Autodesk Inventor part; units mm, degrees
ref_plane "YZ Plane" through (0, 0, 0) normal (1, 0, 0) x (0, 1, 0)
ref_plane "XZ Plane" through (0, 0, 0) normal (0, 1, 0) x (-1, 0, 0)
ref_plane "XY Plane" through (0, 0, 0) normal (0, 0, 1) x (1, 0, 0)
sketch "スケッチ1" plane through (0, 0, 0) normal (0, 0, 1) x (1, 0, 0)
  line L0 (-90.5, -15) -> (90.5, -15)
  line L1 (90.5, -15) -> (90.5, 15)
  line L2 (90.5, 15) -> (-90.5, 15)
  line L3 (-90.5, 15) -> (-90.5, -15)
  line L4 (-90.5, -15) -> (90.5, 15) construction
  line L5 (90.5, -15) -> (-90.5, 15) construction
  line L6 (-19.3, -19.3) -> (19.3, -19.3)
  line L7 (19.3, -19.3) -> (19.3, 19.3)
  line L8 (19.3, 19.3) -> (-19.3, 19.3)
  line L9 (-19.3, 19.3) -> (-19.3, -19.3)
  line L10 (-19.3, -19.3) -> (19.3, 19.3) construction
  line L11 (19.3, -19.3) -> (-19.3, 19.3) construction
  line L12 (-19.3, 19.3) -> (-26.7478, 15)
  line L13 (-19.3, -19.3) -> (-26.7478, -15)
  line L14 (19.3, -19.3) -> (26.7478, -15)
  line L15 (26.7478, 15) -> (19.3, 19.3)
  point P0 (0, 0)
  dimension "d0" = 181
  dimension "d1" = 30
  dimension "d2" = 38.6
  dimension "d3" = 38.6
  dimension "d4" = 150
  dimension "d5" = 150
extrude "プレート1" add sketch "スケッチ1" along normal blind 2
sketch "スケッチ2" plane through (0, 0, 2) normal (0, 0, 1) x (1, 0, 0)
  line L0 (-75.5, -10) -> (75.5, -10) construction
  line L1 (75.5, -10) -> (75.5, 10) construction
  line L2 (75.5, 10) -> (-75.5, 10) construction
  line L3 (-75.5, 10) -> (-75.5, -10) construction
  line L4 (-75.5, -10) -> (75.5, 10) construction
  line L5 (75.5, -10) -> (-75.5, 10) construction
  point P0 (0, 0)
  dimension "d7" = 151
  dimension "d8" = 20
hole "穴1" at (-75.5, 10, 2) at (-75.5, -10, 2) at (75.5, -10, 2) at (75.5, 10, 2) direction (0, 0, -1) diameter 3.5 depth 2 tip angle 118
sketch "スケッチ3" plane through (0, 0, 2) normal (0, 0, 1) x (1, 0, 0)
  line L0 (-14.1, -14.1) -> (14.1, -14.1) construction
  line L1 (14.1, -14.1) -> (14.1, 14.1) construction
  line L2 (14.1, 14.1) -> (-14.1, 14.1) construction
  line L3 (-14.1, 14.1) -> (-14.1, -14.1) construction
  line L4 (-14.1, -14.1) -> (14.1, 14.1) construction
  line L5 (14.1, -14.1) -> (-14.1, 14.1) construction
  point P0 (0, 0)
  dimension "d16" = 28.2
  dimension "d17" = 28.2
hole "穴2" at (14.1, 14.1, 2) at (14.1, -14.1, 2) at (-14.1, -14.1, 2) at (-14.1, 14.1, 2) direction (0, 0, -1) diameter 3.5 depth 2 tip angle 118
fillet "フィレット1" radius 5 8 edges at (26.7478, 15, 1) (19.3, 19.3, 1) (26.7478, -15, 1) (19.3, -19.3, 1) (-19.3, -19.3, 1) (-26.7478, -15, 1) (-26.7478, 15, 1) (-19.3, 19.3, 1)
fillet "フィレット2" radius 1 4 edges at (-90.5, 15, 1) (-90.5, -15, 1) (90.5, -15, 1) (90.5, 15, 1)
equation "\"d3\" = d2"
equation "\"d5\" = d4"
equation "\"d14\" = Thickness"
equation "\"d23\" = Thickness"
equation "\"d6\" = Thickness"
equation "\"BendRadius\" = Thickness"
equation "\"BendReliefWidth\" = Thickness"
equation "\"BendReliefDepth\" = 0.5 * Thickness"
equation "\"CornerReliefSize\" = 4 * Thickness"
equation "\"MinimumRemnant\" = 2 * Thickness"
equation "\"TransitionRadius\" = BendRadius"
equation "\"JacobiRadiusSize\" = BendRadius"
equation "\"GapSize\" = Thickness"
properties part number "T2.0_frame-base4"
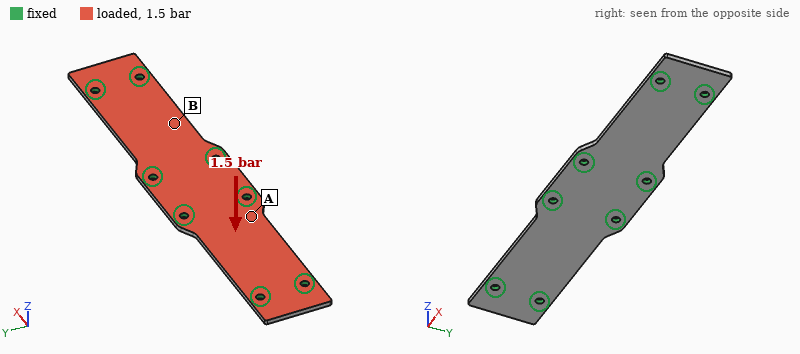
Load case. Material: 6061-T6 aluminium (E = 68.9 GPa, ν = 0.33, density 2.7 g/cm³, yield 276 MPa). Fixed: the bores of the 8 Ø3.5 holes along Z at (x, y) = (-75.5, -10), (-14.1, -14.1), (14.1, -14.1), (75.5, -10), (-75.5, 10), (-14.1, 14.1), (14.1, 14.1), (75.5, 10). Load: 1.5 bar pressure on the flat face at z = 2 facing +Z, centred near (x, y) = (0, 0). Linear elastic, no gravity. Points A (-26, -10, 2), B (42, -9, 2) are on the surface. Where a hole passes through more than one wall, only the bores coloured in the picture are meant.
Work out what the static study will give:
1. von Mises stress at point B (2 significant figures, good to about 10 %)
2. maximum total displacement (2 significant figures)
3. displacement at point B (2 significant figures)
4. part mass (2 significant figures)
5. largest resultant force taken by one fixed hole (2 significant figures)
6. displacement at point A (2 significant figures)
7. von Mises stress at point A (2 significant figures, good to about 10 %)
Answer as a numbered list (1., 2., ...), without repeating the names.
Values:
1. 31 MPa
2. 0.11 mm
3. 0.11 mm
4. 31 g
5. 110 N
6. 0.046 mm
7. 11 MPa
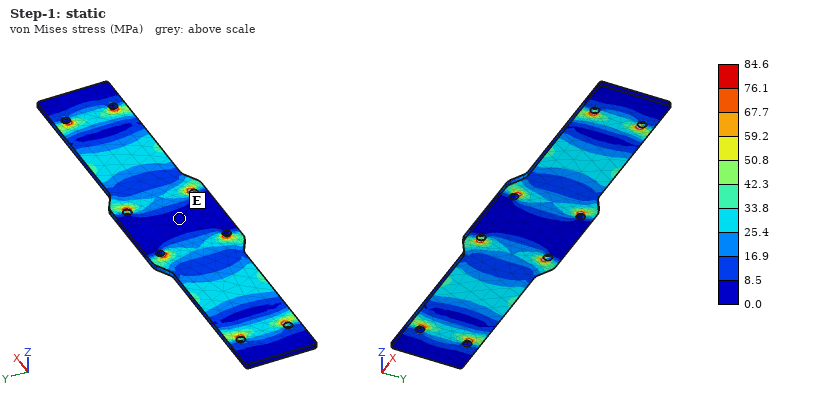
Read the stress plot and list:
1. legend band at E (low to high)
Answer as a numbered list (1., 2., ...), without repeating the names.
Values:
1. 0.0 to 8.5 MPa
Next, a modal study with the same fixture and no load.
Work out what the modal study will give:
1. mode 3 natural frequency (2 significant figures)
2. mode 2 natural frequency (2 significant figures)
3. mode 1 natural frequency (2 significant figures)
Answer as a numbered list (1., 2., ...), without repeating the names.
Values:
1. 4900 Hz
2. 2900 Hz
3. 2900 Hz
